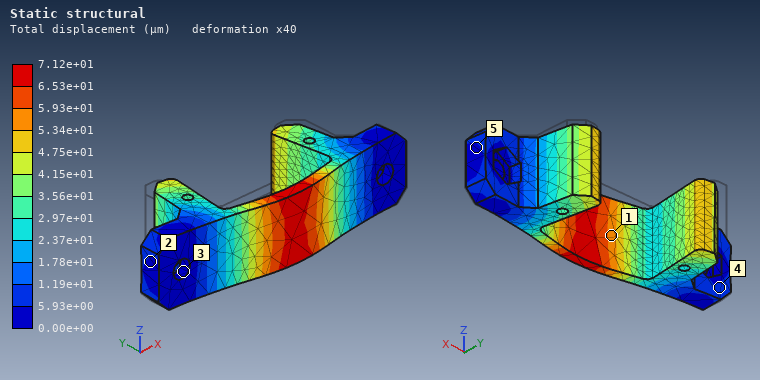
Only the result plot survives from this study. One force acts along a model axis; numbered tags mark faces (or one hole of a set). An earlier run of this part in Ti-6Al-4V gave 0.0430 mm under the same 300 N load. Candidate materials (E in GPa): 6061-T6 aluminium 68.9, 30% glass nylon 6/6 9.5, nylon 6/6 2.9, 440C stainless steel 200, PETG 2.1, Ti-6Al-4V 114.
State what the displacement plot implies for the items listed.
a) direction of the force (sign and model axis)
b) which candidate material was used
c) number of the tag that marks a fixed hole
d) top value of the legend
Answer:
-Y
6061-T6 aluminium
3
7.12e+01 µm
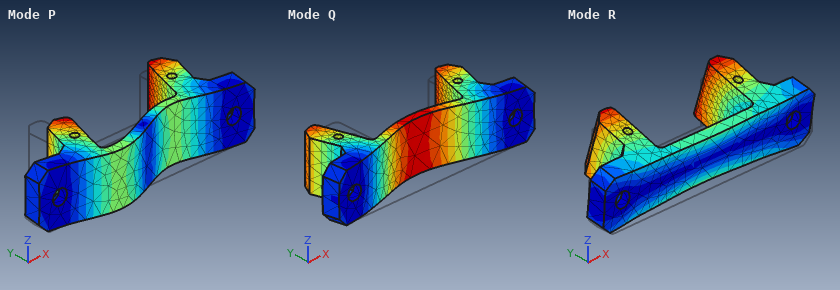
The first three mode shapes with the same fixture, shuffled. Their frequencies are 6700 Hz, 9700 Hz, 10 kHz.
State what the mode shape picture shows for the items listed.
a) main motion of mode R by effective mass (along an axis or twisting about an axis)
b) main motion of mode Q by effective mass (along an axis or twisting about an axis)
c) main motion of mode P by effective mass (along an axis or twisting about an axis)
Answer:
along Z
along Y
along X
